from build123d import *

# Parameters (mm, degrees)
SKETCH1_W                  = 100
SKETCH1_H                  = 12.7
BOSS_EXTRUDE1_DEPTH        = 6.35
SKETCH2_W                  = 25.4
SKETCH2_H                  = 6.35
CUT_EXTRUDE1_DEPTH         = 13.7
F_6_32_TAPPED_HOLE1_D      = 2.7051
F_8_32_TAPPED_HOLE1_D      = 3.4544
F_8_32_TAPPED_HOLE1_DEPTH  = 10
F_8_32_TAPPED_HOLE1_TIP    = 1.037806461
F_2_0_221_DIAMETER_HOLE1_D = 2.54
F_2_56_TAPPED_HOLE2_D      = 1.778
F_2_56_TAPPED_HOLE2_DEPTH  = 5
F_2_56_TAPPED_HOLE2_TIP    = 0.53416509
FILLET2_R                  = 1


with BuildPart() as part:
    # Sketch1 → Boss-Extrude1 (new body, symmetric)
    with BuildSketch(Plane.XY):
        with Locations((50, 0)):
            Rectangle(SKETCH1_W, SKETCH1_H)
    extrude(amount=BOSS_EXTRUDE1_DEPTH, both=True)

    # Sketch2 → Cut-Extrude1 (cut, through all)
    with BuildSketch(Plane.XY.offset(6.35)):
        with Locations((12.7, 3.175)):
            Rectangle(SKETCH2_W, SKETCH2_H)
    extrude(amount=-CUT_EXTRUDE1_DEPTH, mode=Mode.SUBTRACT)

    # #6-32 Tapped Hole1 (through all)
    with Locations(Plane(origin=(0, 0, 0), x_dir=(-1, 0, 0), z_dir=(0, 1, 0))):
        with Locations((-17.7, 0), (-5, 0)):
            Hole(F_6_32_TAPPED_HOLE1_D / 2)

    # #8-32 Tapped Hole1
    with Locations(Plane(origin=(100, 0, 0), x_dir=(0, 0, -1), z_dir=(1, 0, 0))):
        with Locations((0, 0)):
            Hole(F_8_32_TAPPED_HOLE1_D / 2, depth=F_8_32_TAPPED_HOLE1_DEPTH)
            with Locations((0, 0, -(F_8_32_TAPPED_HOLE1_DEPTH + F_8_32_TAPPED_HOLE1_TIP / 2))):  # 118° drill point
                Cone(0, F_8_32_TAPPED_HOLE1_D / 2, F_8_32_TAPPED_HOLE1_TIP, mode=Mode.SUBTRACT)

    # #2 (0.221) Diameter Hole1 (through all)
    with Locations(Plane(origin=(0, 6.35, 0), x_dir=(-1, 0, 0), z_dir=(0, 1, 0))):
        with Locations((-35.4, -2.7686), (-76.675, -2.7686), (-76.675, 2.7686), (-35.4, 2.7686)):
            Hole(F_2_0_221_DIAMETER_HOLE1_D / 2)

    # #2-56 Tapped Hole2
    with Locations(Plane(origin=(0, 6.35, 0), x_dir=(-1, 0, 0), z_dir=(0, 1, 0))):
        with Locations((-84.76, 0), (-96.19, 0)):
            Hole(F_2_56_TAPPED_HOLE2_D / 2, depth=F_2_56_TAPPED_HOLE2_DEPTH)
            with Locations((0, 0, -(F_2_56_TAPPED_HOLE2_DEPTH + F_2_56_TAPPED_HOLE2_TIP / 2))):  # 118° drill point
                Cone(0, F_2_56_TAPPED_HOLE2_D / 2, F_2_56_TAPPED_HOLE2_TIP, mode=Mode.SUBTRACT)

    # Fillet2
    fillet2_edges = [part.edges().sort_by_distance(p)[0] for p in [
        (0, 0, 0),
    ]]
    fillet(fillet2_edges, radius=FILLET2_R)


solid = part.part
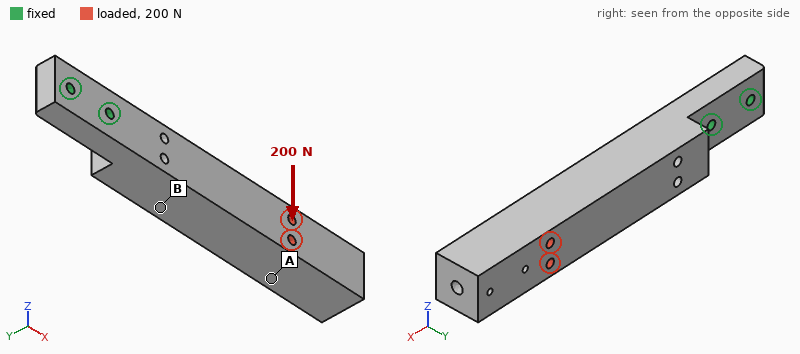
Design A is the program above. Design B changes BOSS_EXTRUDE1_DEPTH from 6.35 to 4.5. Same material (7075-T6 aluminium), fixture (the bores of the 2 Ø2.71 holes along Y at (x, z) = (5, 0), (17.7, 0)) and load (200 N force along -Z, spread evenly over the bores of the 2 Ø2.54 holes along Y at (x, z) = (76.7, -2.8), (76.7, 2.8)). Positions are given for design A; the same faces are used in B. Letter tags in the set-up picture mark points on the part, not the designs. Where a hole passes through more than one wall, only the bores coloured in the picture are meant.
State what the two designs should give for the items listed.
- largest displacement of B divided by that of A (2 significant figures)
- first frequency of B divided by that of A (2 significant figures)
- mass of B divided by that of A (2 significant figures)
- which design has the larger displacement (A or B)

2.6
1.0
0.70
B
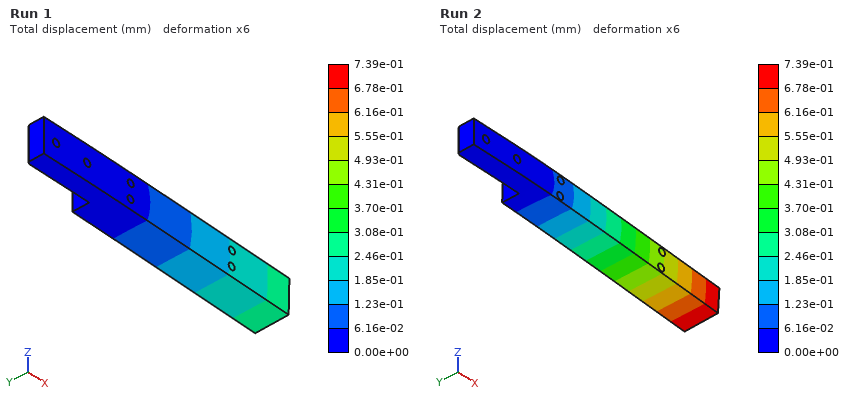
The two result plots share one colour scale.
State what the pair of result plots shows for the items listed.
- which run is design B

Run 2
